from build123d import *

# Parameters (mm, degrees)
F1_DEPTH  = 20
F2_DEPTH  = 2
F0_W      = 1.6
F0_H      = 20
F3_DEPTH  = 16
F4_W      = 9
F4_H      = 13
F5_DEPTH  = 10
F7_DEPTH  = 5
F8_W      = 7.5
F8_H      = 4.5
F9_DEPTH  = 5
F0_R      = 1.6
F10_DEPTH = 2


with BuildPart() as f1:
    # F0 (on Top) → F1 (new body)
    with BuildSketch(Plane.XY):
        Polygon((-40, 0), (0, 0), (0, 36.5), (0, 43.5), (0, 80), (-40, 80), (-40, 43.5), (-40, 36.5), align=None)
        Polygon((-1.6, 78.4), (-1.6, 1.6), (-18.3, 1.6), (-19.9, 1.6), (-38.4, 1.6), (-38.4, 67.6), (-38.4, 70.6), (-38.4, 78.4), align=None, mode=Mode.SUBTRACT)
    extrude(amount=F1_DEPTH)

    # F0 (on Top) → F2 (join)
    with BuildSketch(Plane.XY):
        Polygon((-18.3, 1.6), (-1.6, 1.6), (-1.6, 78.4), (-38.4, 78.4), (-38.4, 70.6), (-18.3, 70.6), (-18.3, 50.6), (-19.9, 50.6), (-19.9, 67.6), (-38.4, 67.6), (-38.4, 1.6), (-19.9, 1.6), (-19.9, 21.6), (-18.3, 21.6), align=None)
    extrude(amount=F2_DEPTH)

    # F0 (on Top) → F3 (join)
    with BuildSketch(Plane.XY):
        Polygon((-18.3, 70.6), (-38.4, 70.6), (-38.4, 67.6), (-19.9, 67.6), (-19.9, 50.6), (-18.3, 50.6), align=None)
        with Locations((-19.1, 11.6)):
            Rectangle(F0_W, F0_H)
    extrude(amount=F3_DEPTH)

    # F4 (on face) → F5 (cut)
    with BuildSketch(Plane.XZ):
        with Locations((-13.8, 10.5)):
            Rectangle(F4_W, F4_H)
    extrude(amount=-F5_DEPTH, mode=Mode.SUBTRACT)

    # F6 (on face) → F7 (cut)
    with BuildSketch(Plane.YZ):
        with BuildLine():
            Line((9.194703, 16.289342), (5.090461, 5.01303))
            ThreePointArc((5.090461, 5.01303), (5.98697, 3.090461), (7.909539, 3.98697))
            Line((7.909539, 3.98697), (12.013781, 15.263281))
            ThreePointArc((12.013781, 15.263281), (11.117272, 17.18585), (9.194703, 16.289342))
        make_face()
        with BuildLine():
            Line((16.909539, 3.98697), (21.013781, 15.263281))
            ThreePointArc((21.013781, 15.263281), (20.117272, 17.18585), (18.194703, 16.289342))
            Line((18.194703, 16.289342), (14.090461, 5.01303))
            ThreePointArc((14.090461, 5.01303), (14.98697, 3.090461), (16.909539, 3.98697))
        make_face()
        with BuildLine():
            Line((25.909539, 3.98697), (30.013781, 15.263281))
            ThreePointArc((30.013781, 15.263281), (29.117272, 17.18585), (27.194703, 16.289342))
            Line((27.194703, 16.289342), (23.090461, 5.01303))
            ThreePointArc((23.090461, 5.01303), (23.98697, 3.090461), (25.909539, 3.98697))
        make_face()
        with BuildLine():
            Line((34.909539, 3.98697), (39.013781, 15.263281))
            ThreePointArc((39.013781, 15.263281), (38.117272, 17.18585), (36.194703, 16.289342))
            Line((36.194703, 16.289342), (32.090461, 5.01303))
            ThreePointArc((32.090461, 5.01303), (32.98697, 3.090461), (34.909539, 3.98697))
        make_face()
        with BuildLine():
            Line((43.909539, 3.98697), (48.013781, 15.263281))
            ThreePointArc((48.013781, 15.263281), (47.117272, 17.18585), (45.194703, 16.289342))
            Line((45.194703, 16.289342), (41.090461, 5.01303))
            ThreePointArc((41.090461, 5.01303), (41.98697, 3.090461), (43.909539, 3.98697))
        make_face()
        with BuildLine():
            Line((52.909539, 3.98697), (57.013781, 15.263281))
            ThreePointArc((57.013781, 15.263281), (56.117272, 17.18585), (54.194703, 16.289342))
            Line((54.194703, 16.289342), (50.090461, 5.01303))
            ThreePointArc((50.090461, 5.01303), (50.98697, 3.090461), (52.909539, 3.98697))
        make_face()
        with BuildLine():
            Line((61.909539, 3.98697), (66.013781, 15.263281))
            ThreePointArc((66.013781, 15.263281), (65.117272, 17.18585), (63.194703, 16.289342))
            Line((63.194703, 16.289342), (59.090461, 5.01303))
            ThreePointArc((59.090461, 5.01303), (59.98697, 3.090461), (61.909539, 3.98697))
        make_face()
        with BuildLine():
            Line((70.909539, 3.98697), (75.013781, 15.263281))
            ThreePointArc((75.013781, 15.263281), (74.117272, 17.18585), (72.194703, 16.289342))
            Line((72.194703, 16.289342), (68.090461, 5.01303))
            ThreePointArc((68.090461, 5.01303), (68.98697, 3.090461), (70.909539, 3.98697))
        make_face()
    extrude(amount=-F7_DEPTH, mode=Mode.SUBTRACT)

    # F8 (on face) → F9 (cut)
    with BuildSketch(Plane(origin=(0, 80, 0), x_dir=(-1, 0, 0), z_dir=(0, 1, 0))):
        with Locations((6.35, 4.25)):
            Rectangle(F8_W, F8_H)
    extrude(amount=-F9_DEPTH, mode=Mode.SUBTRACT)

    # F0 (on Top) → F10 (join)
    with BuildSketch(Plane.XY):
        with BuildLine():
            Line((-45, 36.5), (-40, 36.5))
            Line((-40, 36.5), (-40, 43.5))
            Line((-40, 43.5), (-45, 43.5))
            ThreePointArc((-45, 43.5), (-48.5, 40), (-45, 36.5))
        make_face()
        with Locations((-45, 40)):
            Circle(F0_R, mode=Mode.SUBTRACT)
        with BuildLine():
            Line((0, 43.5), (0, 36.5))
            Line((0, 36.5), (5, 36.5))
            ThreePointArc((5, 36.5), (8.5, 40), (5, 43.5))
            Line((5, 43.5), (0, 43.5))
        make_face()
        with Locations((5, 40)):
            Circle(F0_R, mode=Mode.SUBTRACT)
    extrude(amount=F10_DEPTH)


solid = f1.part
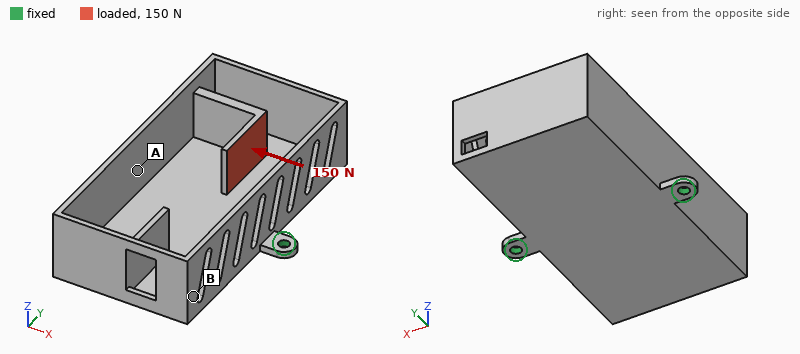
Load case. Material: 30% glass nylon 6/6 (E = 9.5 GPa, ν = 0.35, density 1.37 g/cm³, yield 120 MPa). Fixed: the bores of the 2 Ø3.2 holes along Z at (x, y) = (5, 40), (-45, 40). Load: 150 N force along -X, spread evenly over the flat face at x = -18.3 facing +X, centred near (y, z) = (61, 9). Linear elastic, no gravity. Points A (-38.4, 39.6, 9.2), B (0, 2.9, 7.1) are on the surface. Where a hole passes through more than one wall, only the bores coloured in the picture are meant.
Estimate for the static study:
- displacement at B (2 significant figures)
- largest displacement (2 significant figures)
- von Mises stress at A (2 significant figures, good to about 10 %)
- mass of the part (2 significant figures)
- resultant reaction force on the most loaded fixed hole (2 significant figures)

0.24 mm
0.69 mm
6.6 MPa
19 g
110 N
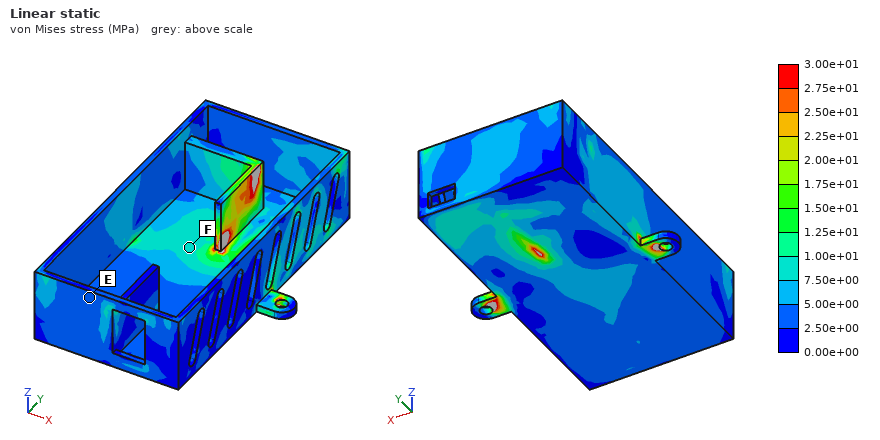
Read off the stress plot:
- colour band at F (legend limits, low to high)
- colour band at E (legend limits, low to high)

7.50e+00 to 1.00e+01 MPa
2.50e+00 to 5.00e+00 MPa
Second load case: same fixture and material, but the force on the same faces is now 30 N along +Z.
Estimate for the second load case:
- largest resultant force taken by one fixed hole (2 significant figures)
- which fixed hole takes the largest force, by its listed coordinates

16 N
(5, 40)
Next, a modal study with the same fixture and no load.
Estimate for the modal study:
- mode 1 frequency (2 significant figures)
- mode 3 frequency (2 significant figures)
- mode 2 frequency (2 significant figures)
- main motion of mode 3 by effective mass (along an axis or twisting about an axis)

240 Hz
1300 Hz
800 Hz
along Z
